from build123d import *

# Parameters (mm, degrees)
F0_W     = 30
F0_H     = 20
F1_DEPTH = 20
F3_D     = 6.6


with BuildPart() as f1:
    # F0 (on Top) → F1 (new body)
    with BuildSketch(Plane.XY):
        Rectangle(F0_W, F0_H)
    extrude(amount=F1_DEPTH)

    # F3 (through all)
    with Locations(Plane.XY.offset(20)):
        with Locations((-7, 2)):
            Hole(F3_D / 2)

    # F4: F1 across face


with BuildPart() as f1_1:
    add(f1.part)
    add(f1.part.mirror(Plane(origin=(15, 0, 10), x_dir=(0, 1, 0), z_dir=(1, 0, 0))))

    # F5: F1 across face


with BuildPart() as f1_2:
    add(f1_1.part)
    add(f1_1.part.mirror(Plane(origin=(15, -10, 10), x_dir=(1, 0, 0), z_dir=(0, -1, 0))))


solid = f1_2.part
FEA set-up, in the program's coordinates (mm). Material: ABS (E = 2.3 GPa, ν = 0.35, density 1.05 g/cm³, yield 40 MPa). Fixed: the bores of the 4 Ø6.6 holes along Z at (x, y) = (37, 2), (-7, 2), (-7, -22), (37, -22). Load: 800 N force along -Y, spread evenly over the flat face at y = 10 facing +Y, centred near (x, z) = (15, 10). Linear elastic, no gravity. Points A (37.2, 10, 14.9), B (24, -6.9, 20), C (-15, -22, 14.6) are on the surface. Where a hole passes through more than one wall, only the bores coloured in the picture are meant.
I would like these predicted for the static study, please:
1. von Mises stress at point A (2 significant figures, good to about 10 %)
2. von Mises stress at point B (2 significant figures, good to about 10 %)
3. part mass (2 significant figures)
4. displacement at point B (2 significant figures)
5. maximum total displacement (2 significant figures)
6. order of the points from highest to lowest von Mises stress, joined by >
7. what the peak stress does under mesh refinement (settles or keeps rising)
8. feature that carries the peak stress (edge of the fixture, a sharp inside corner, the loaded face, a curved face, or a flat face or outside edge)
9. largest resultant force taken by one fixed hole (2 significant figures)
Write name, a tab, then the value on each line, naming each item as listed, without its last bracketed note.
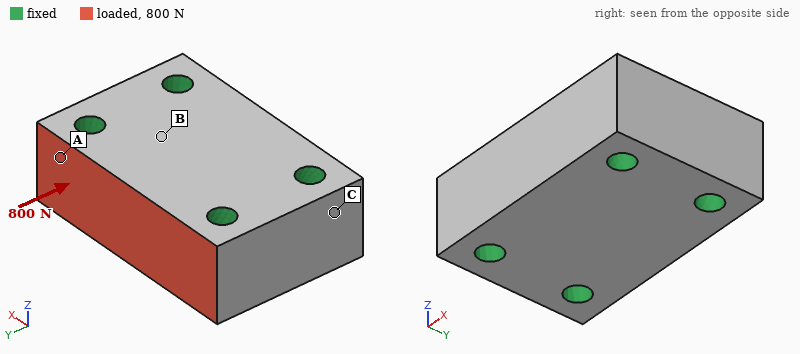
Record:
von Mises stress at point A	1.2 MPa
von Mises stress at point B	0.53 MPa
part mass	48 g
displacement at point B	4.3 µm
maximum total displacement	9.3 µm
order of the points from highest to lowest von Mises stress, joined by >	A > B > C
what the peak stress does under mesh refinement	keeps rising
feature that carries the peak stress	edge of the fixture
largest resultant force taken by one fixed hole	300 N
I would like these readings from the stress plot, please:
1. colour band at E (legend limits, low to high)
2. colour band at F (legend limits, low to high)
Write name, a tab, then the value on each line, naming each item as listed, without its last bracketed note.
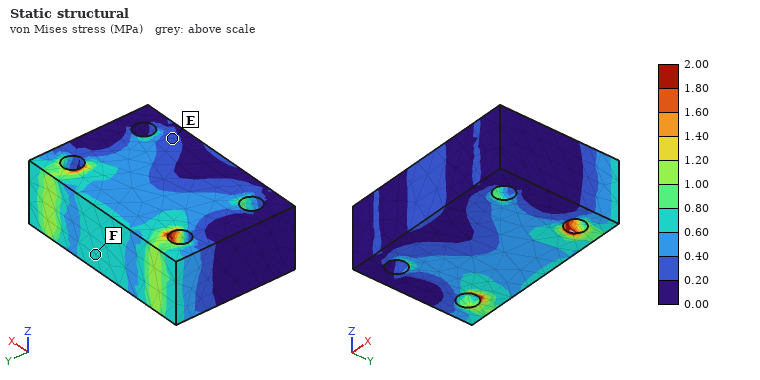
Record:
colour band at E	0.20 to 0.40 MPa
colour band at F	0.60 to 0.80 MPa
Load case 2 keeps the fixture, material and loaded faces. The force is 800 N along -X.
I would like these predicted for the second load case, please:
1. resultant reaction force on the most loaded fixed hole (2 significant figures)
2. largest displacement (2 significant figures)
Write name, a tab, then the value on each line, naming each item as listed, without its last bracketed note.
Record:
resultant reaction force on the most loaded fixed hole	390 N
largest displacement	11 µm
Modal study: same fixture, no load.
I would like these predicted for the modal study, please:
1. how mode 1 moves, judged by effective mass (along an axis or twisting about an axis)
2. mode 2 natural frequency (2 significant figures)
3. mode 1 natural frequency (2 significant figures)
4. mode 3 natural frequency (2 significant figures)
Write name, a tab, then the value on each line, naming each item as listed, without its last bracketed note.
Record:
how mode 1 moves, judged by effective mass	along Z
mode 2 natural frequency	9600 Hz
mode 1 natural frequency	8400 Hz
mode 3 natural frequency	9700 Hz
